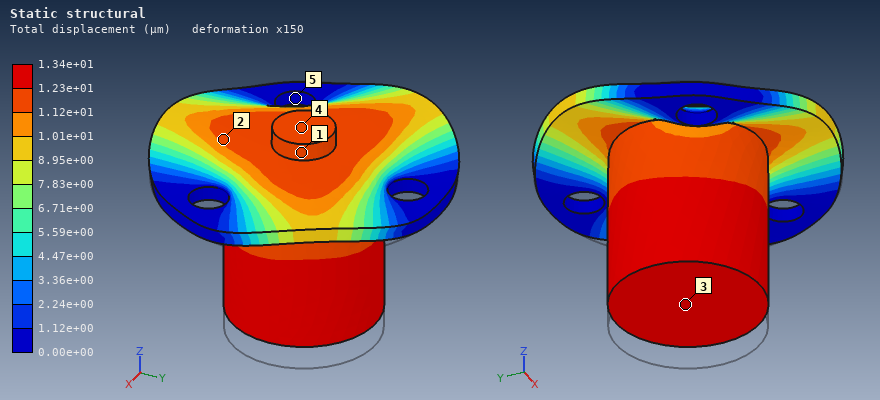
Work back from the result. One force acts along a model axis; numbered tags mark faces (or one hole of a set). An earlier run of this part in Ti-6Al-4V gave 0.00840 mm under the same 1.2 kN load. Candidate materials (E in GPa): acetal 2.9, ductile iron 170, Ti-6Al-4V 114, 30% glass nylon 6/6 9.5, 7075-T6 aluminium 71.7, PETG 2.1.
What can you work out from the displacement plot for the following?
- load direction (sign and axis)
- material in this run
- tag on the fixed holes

+Z
7075-T6 aluminium
5
